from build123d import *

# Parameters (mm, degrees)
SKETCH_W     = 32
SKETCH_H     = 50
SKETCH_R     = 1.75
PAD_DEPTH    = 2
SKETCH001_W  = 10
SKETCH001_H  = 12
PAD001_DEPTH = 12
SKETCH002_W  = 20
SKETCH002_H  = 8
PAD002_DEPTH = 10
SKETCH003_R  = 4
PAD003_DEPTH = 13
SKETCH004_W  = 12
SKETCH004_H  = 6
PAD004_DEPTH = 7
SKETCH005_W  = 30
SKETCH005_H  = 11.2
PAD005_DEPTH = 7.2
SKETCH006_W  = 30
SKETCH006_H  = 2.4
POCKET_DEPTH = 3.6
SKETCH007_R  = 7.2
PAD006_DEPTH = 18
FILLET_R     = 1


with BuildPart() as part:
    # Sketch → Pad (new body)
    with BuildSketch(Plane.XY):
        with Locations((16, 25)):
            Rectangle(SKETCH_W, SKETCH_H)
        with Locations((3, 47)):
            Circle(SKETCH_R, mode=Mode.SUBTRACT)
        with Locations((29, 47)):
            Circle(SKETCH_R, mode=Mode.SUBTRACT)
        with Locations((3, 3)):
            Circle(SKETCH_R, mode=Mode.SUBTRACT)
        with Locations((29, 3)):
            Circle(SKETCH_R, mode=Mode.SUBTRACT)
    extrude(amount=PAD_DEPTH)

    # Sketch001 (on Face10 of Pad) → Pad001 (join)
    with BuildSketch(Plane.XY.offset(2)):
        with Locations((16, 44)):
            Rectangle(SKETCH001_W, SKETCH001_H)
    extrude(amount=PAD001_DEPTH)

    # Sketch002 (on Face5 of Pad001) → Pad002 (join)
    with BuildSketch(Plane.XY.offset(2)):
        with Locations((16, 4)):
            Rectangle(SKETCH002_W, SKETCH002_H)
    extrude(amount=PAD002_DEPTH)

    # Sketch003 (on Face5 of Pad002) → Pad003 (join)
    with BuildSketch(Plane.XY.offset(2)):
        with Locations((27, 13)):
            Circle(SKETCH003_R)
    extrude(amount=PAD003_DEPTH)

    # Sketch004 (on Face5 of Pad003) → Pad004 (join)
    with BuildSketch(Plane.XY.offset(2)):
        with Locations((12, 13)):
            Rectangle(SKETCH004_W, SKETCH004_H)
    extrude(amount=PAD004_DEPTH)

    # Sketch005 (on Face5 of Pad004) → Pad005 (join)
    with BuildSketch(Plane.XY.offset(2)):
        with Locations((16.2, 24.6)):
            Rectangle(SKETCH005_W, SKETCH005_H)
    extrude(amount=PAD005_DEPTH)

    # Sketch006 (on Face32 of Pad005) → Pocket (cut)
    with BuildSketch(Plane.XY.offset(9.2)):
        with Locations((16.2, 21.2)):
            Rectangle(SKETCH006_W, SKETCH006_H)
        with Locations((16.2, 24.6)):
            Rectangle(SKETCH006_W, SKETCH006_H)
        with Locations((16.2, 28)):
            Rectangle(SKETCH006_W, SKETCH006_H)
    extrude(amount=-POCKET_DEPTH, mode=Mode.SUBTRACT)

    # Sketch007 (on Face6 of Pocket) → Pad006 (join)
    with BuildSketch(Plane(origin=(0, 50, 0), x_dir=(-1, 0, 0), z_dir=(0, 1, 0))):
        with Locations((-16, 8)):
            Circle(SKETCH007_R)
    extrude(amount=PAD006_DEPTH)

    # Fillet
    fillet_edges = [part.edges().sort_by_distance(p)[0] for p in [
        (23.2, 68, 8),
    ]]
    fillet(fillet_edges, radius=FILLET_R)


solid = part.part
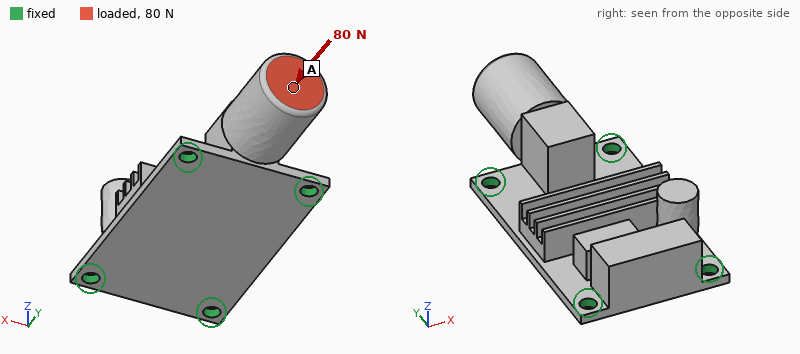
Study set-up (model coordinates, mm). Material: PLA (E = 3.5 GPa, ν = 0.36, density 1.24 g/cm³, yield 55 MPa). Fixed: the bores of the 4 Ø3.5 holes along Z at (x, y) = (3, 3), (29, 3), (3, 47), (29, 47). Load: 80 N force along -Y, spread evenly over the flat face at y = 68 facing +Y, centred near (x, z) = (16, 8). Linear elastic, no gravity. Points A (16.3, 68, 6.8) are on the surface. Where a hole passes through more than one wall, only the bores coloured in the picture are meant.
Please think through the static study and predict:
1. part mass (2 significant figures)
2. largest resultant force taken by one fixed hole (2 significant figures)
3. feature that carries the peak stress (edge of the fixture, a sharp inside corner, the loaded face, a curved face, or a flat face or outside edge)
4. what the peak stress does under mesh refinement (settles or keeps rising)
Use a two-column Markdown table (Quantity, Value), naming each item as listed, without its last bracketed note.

| Quantity | Value |
|---|---|
| part mass | 15 g |
| largest resultant force taken by one fixed hole | 30 N |
| feature that carries the peak stress | edge of the fixture |
| what the peak stress does under mesh refinement | keeps rising |
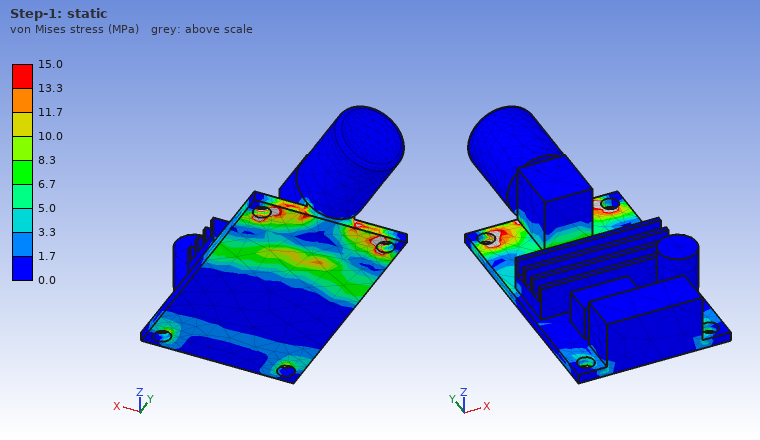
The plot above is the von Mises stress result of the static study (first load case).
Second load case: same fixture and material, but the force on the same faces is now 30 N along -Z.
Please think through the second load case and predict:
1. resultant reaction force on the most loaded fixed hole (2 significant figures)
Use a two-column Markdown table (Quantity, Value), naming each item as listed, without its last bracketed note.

| Quantity | Value |
|---|---|
| resultant reaction force on the most loaded fixed hole | 27 N |
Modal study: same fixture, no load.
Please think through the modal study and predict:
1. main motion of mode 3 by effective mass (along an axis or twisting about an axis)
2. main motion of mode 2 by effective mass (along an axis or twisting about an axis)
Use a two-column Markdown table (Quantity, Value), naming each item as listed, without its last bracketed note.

| Quantity | Value |
|---|---|
| main motion of mode 3 by effective mass | along X |
| main motion of mode 2 by effective mass | along Z |
